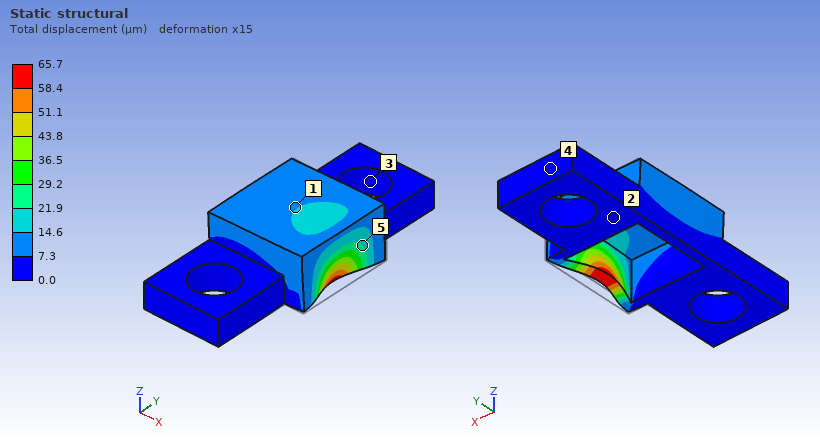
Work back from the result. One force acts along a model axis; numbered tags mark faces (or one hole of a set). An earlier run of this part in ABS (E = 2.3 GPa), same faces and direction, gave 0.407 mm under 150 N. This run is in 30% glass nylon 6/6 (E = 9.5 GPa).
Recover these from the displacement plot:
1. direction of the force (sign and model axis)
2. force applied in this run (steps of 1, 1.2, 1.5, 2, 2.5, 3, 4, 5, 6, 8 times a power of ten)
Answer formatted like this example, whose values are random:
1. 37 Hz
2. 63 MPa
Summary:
1. -X
2. 100 N
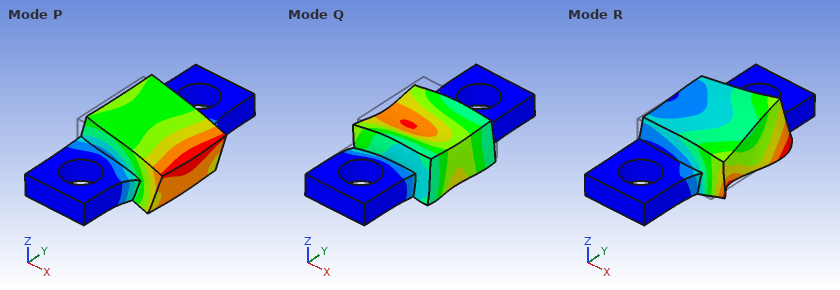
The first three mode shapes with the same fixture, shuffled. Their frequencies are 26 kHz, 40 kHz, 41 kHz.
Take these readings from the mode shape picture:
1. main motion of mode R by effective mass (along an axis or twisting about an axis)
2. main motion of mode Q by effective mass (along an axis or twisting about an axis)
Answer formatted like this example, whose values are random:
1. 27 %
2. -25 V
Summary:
1. along Y
2. along Z
